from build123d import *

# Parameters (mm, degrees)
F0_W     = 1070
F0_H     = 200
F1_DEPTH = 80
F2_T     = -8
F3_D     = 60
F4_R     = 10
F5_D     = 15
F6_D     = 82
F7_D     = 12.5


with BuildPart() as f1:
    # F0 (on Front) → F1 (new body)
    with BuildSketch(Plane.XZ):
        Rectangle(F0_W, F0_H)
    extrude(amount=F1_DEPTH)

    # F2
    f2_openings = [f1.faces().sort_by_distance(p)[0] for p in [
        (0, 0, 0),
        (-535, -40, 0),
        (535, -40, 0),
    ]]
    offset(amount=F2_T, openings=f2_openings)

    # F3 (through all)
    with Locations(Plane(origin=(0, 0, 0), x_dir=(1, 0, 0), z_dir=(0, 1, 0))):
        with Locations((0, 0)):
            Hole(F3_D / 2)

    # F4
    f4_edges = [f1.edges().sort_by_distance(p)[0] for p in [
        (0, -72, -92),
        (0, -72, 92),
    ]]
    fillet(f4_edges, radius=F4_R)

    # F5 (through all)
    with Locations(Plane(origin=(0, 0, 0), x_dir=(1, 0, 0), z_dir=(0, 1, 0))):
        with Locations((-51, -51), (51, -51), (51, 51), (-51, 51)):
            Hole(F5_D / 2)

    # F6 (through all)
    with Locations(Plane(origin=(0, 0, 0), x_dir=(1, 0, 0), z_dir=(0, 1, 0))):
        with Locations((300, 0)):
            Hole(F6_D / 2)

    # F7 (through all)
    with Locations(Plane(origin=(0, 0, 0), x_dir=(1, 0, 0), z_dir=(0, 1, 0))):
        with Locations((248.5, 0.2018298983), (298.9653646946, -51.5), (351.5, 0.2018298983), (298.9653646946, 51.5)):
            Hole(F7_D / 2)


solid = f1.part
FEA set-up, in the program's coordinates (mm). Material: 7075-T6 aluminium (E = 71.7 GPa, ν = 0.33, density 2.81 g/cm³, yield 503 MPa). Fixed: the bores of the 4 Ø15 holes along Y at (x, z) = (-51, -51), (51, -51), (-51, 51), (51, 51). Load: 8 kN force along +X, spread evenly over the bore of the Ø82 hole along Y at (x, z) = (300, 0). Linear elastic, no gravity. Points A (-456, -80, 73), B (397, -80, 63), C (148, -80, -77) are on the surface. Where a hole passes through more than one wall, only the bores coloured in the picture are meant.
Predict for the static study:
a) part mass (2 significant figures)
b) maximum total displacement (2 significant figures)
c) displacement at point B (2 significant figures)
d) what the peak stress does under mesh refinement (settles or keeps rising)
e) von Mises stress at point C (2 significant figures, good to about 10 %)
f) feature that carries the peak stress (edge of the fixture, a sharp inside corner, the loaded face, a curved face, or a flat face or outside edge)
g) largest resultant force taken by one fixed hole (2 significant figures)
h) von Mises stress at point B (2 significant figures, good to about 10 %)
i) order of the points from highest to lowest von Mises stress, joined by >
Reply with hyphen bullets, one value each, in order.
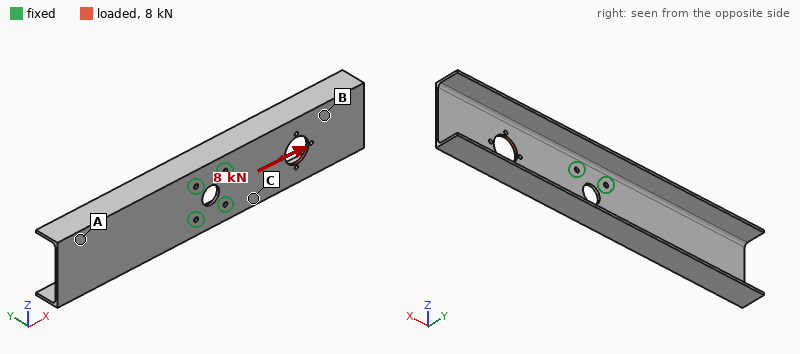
- 8.2 kg
- 0.12 mm
- 0.069 mm
- keeps rising
- 4.5 MPa
- a sharp inside corner
- 3.3 kN
- 1.7 MPa
- C > B > A
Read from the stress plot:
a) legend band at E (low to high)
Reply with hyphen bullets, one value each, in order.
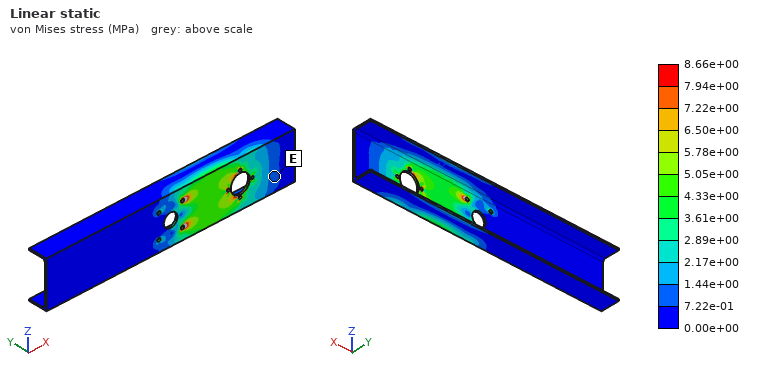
- 7.22e-01 to 1.44e+00 MPa
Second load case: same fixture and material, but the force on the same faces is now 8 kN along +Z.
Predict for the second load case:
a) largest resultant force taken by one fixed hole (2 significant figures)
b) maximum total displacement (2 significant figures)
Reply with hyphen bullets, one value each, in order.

- 12 kN
- 0.58 mm
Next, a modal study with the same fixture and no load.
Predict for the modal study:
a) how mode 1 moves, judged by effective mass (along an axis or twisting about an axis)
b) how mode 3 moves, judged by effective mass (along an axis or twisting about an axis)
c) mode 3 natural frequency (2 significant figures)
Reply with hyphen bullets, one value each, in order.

- twisting about Z
- along Y
- 210 Hz
